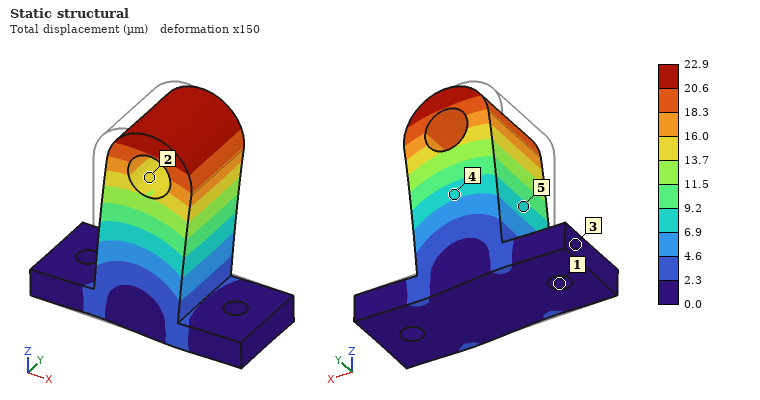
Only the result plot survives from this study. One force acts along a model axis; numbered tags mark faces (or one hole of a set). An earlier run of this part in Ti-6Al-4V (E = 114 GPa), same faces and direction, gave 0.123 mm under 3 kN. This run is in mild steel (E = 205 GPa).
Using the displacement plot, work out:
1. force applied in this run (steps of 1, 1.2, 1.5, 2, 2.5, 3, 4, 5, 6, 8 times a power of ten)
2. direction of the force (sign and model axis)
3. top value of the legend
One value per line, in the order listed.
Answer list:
1 kN
+X
22.9 µm
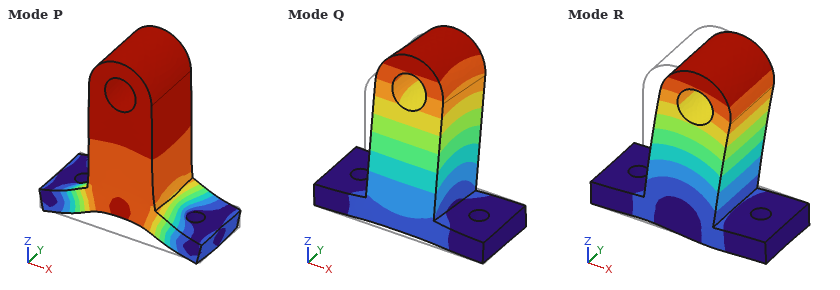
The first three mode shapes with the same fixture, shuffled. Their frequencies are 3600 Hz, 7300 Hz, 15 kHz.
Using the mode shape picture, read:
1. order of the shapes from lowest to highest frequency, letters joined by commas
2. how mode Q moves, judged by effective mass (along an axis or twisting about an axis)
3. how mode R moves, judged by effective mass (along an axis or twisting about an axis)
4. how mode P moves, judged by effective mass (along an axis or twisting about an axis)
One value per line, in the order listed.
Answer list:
Q, R, P
along Y
along X
along Z
